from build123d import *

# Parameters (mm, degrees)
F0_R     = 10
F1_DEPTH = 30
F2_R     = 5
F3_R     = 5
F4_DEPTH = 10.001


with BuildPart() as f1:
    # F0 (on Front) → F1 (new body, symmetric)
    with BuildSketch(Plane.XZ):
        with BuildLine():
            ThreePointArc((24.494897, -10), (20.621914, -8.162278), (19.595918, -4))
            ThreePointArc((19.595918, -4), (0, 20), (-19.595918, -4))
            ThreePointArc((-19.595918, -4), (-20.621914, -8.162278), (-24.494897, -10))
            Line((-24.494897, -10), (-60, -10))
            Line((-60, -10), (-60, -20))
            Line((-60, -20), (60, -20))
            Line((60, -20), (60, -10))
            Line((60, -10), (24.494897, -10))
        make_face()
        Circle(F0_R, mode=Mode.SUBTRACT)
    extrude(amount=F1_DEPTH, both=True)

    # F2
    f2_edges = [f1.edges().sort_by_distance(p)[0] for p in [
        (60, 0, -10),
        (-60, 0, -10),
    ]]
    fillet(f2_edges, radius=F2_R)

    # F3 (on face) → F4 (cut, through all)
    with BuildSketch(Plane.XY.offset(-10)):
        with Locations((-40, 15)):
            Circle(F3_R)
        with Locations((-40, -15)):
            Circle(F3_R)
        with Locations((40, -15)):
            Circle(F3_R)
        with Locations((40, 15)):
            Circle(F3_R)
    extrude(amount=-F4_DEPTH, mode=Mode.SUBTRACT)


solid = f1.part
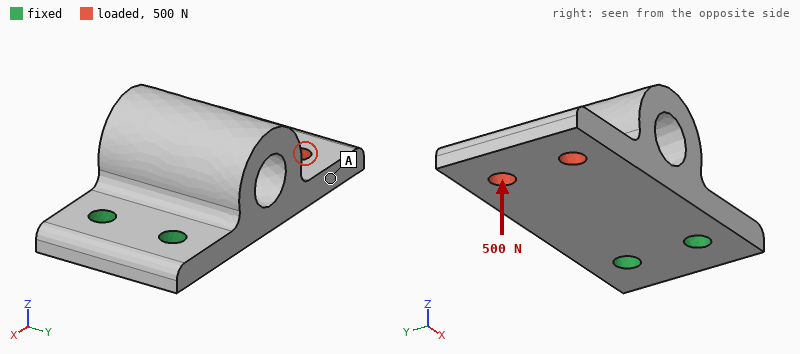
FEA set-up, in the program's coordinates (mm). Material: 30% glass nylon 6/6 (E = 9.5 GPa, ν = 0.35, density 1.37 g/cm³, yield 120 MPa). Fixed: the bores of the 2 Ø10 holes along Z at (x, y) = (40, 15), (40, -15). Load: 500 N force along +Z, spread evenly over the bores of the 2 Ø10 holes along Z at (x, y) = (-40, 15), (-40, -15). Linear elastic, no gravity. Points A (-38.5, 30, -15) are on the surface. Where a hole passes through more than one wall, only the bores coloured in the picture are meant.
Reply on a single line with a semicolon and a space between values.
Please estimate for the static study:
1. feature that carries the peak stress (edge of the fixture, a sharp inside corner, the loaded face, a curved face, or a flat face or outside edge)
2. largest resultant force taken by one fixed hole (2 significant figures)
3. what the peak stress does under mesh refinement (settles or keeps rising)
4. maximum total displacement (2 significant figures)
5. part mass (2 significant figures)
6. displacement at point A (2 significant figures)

edge of the fixture; 250 N; keeps rising; 1.5 mm; 150 g; 1.1 mm
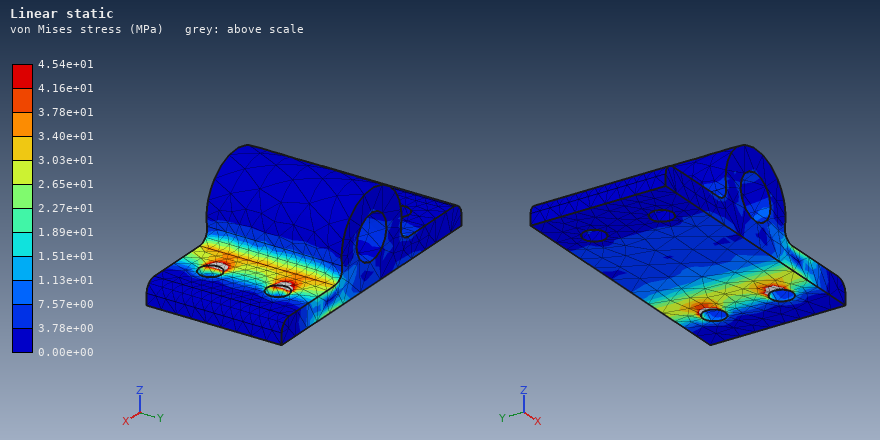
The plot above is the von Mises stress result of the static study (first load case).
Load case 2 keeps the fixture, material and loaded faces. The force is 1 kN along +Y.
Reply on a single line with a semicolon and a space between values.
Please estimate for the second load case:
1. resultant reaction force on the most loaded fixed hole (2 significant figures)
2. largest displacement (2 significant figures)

2.2 kN; 0.20 mm
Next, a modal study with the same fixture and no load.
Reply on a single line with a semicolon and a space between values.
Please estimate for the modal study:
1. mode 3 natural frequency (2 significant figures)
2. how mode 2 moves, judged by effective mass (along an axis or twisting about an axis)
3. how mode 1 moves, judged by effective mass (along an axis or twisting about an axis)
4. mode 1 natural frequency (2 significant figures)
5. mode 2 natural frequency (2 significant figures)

1900 Hz; along Y; along Z; 470 Hz; 1700 Hz
